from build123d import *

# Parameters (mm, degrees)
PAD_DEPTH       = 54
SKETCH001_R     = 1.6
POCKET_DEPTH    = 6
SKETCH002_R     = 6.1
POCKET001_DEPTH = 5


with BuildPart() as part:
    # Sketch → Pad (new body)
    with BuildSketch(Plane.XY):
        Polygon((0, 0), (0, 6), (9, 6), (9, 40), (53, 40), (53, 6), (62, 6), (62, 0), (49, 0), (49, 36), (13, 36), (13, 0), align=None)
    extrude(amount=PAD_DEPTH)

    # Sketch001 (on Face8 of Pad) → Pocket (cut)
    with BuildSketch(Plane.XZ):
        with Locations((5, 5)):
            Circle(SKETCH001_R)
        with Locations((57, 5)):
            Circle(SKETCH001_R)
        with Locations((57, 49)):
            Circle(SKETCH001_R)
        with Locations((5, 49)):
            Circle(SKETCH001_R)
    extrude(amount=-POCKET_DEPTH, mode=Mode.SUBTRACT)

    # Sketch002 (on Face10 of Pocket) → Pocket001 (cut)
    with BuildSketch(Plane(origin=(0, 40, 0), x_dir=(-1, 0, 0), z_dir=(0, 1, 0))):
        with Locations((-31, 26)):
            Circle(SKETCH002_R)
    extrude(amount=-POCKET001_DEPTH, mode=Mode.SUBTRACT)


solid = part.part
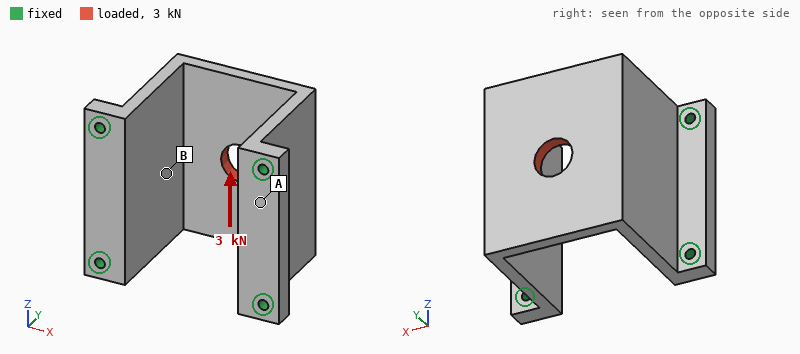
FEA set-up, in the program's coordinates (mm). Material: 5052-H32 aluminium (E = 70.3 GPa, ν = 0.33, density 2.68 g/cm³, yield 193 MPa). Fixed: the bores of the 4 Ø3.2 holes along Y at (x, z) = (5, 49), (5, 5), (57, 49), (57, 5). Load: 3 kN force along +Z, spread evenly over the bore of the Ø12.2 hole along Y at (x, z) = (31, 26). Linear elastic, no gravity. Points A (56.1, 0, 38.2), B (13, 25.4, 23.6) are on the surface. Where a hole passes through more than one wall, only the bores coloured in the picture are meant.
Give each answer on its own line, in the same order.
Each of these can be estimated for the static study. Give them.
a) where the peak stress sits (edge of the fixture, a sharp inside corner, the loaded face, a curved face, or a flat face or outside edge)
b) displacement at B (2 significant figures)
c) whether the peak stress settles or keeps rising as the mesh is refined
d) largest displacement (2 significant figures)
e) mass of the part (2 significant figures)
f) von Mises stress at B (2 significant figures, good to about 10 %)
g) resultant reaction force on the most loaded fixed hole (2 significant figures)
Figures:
edge of the fixture
17 µm
keeps rising
36 µm
81 g
21 MPa
1.4 kN
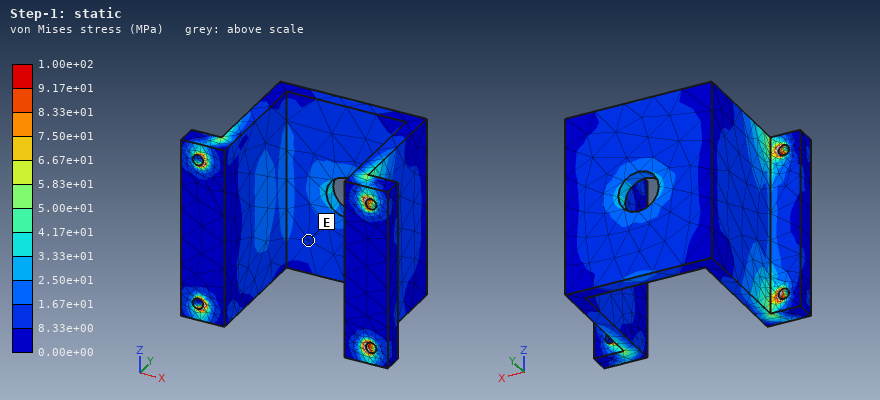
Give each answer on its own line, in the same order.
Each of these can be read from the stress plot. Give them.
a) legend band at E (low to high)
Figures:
8.33e+00 to 1.67e+01 MPa
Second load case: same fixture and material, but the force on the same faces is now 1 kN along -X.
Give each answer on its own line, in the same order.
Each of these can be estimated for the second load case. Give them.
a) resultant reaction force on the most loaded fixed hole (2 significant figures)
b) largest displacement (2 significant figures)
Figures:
360 N
0.13 mm
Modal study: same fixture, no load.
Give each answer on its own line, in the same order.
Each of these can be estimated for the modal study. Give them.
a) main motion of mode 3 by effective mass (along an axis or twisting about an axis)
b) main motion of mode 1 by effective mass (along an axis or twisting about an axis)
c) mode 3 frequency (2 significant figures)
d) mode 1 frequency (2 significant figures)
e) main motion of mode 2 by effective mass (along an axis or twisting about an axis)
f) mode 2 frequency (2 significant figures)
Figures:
along Z
along X
7900 Hz
2300 Hz
twisting about Y
7000 Hz
